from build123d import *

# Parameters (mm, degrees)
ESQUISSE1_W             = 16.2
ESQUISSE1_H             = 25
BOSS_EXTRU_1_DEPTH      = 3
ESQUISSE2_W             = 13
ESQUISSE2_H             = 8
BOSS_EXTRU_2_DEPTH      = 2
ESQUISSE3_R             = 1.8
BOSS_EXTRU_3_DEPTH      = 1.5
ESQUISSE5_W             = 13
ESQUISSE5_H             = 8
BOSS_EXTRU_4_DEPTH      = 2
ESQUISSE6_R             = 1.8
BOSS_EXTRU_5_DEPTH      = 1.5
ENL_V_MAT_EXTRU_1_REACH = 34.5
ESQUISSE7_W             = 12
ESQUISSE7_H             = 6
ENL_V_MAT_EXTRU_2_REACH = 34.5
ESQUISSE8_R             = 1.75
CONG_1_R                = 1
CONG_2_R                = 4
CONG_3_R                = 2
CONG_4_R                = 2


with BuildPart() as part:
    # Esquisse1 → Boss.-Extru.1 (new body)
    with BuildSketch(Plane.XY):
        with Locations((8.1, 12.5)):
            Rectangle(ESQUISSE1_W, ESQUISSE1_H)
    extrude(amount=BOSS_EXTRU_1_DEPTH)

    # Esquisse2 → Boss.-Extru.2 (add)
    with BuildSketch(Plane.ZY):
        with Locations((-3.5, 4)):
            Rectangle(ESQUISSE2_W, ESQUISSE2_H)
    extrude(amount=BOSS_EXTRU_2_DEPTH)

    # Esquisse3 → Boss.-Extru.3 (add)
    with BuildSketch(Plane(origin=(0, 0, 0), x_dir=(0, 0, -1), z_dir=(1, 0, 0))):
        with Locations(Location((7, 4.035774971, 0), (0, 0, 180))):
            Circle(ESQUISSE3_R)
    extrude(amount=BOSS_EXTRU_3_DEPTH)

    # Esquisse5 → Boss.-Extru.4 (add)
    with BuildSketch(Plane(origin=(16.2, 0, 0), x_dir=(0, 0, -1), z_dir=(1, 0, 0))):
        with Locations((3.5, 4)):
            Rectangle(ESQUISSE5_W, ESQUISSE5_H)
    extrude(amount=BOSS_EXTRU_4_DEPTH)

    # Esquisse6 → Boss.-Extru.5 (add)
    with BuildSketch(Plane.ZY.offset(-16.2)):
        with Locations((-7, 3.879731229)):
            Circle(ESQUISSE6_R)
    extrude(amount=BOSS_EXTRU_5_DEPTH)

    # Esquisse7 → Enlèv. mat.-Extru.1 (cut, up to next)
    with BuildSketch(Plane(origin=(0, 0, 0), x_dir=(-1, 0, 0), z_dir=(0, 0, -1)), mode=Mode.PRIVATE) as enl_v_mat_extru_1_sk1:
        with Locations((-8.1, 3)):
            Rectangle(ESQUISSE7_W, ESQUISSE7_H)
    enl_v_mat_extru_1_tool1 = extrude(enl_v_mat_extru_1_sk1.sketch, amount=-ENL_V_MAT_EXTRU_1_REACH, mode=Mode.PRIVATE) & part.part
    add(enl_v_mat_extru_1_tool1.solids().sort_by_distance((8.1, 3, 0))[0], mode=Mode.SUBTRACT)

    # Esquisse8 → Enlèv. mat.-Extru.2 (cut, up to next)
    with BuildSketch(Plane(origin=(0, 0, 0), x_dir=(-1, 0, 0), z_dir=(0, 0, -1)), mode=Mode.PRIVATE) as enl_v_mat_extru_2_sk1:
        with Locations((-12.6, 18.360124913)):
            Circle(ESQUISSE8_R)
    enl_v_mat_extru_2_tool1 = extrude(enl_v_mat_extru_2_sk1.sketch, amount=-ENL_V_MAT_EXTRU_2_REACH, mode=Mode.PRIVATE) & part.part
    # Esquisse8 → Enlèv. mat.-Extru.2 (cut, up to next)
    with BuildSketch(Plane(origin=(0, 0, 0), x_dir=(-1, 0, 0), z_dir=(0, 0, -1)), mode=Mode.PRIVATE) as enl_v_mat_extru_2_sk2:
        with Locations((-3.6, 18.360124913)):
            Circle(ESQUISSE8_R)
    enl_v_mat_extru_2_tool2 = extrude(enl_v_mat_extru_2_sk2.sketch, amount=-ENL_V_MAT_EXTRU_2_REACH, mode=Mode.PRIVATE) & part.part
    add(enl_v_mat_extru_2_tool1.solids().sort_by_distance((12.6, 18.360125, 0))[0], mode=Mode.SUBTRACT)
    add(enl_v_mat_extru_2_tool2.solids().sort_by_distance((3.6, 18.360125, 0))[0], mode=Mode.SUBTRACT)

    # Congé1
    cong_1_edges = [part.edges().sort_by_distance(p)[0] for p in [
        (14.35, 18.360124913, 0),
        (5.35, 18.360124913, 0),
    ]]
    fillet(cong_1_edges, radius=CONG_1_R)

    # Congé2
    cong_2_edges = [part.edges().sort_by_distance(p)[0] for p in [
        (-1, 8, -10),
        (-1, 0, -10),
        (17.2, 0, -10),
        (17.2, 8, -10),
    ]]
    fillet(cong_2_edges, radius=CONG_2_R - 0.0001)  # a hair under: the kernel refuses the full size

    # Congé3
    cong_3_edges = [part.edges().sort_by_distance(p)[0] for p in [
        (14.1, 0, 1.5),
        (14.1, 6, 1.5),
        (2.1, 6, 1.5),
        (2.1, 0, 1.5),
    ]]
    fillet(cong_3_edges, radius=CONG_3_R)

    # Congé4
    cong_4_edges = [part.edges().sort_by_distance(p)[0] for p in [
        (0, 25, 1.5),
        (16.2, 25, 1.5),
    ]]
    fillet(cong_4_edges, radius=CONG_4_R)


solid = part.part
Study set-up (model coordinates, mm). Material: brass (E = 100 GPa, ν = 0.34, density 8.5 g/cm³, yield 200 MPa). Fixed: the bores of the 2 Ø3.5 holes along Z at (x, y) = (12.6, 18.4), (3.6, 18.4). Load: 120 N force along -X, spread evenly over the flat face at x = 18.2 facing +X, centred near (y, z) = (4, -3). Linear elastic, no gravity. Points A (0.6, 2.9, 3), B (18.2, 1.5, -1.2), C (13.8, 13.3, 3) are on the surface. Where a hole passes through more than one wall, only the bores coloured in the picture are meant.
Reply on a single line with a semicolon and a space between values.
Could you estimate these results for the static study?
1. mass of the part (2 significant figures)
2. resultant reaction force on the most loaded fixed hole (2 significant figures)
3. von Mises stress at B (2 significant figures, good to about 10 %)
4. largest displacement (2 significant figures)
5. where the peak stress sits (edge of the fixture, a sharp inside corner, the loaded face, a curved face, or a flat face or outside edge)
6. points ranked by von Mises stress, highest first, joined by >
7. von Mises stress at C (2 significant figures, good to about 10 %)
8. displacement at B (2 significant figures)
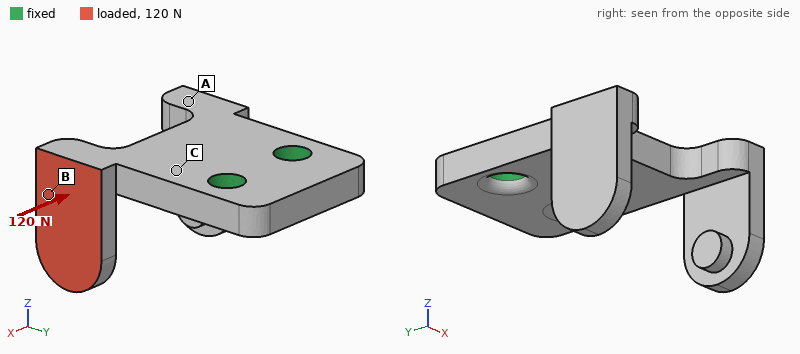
11 g; 180 N; 50 MPa; 83 µm; a curved face; B > C > A; 32 MPa; 32 µm
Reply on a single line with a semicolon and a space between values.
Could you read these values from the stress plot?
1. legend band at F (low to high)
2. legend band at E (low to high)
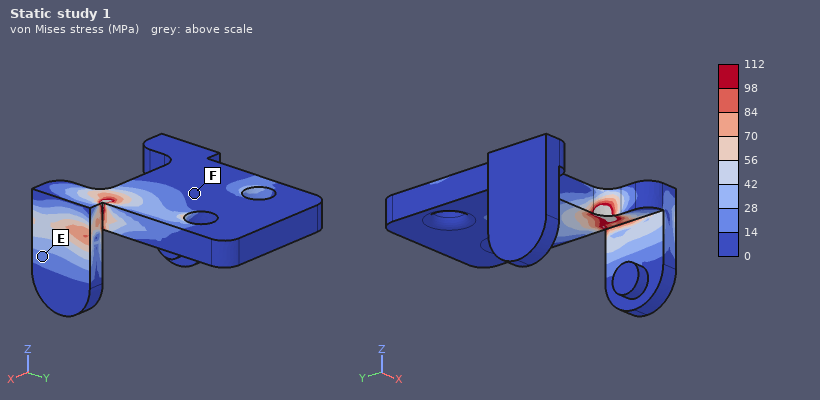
0 to 14 MPa; 14 to 28 MPa
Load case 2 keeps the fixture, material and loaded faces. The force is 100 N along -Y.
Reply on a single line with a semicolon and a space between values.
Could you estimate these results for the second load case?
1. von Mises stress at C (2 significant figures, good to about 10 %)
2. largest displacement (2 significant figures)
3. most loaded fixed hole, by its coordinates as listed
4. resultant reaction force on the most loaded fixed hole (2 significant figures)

18 MPa; 57 µm; (12.6, 18.4); 150 N
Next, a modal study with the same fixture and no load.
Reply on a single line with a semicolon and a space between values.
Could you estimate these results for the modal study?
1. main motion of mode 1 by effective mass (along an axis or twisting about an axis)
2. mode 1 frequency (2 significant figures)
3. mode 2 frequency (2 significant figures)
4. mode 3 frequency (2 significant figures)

along Z; 3500 Hz; 4100 Hz; 5600 Hz
